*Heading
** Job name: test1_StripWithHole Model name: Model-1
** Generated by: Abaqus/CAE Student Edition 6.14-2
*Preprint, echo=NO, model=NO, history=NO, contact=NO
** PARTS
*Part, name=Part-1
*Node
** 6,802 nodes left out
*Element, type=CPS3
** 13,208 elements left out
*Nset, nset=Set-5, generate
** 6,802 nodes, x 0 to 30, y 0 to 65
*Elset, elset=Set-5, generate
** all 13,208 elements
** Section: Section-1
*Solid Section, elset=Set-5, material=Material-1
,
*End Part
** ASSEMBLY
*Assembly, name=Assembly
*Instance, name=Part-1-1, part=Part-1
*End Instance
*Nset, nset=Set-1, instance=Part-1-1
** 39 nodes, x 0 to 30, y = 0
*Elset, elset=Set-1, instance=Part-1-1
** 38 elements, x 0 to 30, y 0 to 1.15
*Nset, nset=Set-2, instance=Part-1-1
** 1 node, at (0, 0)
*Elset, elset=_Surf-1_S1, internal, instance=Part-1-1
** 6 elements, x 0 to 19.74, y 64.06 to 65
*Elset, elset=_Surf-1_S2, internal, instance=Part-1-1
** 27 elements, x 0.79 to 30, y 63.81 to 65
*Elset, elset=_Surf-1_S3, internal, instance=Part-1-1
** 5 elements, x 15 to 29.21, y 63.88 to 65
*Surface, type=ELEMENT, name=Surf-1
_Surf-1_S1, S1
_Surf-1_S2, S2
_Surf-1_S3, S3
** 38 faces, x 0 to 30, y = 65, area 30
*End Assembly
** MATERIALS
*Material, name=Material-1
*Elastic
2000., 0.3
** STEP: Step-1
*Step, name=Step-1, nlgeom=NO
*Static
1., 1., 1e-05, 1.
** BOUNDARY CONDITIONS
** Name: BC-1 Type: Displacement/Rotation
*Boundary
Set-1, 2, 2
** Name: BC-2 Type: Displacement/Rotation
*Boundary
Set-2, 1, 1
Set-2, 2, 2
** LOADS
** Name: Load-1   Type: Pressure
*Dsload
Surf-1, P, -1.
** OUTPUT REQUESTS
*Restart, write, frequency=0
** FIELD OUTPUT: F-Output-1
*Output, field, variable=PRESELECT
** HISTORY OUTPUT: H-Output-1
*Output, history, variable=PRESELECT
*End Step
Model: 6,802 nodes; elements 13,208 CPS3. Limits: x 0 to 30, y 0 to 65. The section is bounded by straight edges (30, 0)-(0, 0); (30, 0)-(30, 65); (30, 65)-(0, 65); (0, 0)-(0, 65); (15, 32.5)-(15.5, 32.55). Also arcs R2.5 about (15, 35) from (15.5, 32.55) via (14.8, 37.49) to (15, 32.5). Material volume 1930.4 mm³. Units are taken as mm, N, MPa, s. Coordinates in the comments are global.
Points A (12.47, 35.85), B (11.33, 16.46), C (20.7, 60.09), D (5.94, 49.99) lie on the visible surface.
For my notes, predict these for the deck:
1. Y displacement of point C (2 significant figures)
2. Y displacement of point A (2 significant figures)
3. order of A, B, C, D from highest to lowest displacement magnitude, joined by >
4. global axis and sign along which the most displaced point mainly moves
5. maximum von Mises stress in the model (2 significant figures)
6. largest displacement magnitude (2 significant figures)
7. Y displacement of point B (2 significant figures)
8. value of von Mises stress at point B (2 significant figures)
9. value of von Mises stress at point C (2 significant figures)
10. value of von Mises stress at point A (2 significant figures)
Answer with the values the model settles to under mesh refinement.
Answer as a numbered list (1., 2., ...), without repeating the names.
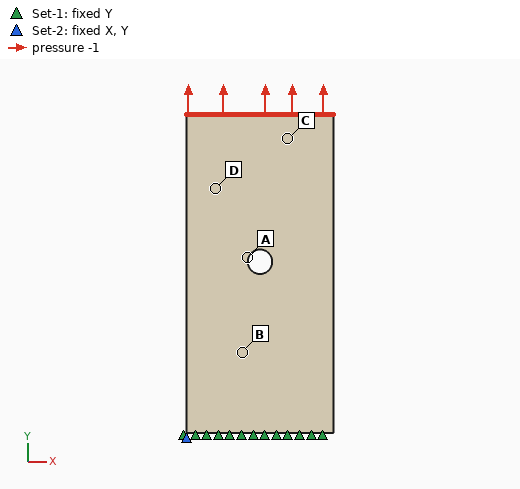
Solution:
1. 0.031 mm
2. 0.019 mm
3. C > D > A > B
4. +Y
5. 3.1 MPa
6. 0.034 mm
7. 0.0081 mm
8. 0.97 MPa
9. 0.99 MPa
10. 2.3 MPa
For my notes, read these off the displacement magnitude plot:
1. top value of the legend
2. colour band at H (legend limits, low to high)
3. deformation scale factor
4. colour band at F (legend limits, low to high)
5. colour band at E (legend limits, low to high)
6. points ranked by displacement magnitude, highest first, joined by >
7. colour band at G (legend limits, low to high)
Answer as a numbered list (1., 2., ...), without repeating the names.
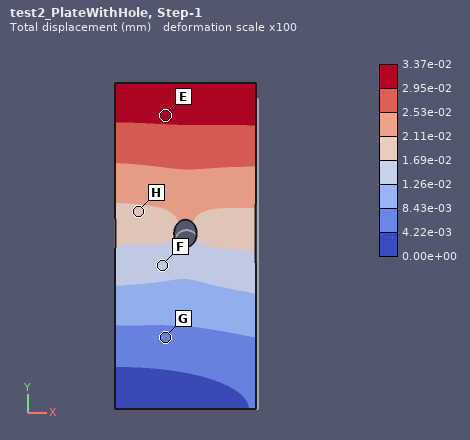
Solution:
1. 3.37e-02 mm
2. 1.69e-02 to 2.11e-02 mm
3. 100
4. 1.26e-02 to 1.69e-02 mm
5. 2.95e-02 to 3.37e-02 mm
6. E > H > F > G
7. 4.22e-03 to 8.43e-03 mm
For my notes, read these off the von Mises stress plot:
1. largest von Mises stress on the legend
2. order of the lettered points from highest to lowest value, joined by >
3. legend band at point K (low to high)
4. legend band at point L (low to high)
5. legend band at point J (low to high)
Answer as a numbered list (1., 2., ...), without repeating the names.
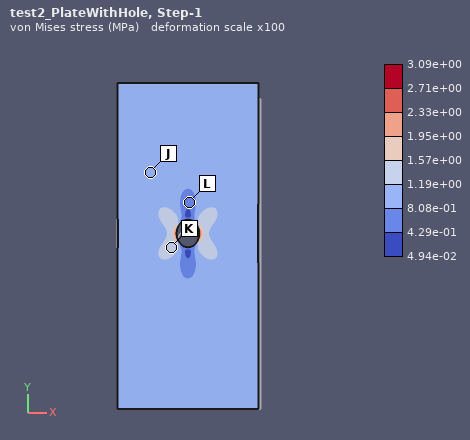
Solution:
1. 3.09e+00 MPa
2. K > J > L
3. 1.19e+00 to 1.57e+00 MPa
4. 4.29e-01 to 8.08e-01 MPa
5. 8.08e-01 to 1.19e+00 MPa
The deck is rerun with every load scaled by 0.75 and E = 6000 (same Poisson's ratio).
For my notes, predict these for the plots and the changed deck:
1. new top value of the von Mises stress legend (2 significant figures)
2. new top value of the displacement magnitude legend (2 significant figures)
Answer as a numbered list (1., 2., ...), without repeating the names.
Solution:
1. 2.3 MPa
2. 0.0084 mm
